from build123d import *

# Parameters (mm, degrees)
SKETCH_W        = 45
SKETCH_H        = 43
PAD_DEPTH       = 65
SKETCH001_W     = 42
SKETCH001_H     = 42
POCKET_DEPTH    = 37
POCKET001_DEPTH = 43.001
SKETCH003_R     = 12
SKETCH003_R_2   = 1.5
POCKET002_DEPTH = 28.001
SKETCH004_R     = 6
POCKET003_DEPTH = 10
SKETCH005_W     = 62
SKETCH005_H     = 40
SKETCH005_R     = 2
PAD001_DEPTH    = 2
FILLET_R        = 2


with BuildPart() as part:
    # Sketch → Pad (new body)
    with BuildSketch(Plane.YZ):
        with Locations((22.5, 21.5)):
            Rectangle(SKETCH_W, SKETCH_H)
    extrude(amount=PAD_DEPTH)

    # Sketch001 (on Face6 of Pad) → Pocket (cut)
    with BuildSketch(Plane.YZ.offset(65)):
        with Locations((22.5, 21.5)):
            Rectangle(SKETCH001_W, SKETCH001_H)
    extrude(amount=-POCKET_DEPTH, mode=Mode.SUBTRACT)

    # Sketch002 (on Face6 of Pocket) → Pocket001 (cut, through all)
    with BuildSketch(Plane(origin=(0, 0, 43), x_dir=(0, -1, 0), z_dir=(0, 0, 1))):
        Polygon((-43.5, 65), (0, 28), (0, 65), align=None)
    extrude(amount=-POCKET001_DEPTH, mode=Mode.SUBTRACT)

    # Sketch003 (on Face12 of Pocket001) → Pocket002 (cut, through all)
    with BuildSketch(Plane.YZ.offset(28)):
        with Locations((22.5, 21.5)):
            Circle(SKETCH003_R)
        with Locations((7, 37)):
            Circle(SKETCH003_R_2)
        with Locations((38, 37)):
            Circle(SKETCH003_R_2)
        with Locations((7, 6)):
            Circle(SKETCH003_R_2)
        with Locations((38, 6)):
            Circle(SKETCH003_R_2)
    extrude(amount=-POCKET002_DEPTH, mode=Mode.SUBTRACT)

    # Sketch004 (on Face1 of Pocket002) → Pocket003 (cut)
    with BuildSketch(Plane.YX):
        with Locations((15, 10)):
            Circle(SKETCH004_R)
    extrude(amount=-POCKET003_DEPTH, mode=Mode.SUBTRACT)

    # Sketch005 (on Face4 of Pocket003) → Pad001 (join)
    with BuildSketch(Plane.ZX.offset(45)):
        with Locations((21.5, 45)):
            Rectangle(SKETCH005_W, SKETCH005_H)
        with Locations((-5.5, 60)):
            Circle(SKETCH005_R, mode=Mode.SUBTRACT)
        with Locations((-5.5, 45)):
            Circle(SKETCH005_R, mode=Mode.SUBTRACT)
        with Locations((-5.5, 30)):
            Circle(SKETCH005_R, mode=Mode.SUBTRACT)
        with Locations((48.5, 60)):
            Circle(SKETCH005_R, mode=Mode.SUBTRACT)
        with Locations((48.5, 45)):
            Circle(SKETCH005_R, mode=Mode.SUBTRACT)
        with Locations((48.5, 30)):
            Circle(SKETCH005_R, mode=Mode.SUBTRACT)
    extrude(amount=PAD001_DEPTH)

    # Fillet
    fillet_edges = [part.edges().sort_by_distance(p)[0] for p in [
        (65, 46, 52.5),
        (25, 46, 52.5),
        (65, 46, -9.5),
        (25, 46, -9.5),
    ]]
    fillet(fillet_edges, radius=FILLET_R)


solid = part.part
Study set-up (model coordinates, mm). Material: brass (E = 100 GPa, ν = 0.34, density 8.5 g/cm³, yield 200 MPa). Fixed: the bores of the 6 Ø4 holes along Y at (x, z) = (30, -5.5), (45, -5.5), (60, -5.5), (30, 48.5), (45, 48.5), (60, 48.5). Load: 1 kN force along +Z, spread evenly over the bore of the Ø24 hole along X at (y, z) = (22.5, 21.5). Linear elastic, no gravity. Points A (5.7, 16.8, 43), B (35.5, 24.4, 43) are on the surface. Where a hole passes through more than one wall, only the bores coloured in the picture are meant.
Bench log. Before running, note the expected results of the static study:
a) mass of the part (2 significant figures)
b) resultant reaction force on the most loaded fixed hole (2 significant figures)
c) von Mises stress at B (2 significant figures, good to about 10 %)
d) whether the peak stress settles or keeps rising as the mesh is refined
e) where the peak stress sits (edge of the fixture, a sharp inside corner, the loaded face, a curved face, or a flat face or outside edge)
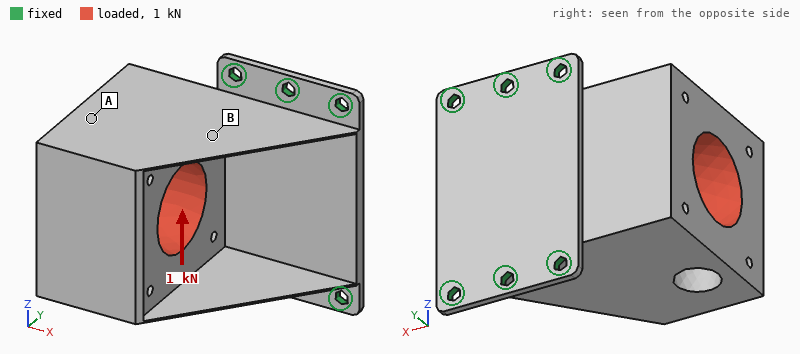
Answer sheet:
400 g
520 N
16 MPa
keeps rising
edge of the fixture
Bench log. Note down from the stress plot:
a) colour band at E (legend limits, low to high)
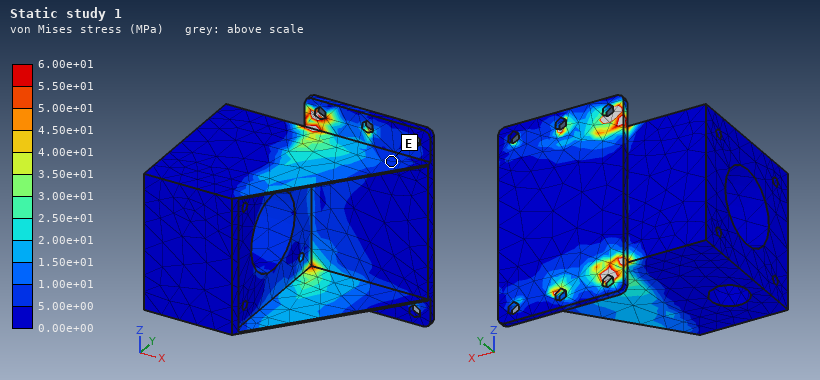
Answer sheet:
5.00e+00 to 1.00e+01 MPa
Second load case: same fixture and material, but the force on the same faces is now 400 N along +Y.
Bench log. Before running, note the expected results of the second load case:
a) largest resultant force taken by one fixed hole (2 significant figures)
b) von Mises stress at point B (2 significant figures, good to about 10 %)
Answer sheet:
340 N
13 MPa
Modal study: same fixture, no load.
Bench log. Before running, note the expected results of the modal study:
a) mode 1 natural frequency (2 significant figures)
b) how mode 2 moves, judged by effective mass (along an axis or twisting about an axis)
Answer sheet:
830 Hz
along Z
